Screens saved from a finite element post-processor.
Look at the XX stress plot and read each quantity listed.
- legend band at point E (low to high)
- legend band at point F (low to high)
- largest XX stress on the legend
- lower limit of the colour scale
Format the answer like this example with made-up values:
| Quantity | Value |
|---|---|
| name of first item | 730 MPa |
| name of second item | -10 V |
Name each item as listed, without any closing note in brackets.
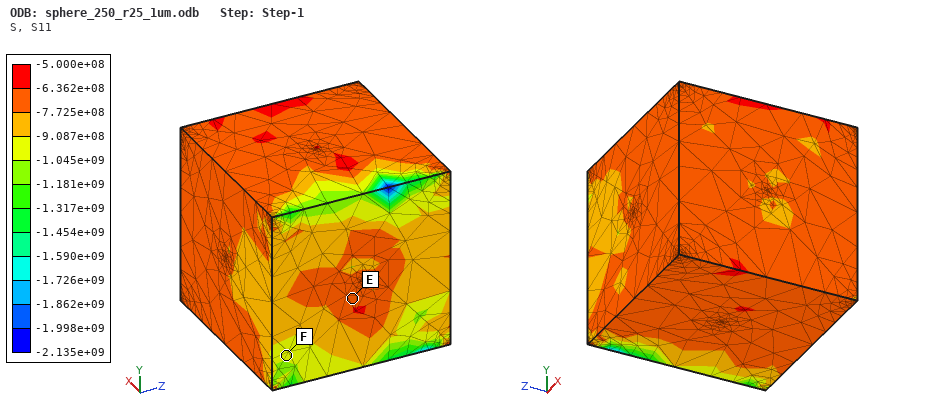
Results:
| Quantity | Value |
|---|---|
| legend band at point E | -7.725e+08 to -6.362e+08 |
| legend band at point F | -1.045e+09 to -9.087e+08 |
| largest XX stress on the legend | -5.000e+08 |
| lower limit of the colour scale | -2.135e+09 |
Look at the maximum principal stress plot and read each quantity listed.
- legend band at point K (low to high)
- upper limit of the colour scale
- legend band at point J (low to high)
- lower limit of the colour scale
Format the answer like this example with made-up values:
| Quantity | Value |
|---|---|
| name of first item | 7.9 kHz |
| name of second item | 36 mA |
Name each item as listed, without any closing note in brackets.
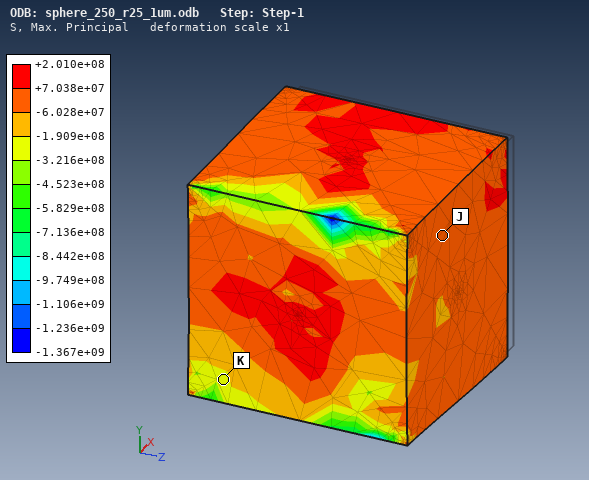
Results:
| Quantity | Value |
|---|---|
| legend band at point K | -3.216e+08 to -1.909e+08 |
| upper limit of the colour scale | +2.010e+08 |
| legend band at point J | -6.028e+07 to +7.038e+07 |
| lower limit of the colour scale | -1.367e+09 |
